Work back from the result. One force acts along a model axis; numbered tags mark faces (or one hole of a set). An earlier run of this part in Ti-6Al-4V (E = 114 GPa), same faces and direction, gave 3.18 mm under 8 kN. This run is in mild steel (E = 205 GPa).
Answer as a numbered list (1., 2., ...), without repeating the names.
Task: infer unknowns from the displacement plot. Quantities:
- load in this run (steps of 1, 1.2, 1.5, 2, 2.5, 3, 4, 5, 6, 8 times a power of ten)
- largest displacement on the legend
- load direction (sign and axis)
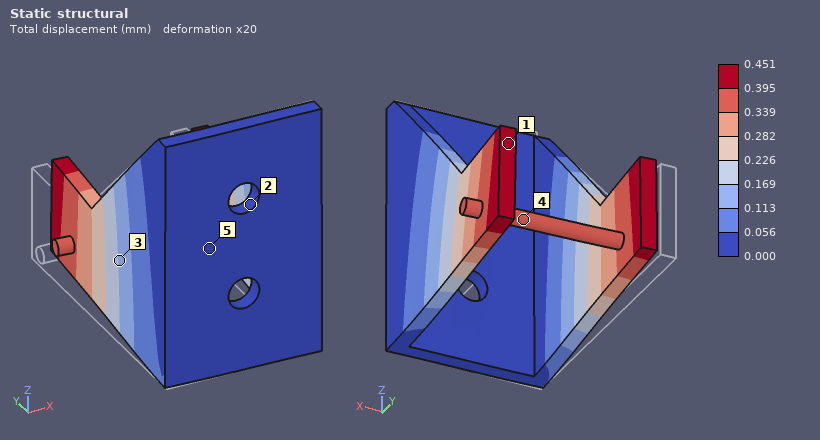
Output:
1. 2 kN
2. 0.451 mm
3. +X
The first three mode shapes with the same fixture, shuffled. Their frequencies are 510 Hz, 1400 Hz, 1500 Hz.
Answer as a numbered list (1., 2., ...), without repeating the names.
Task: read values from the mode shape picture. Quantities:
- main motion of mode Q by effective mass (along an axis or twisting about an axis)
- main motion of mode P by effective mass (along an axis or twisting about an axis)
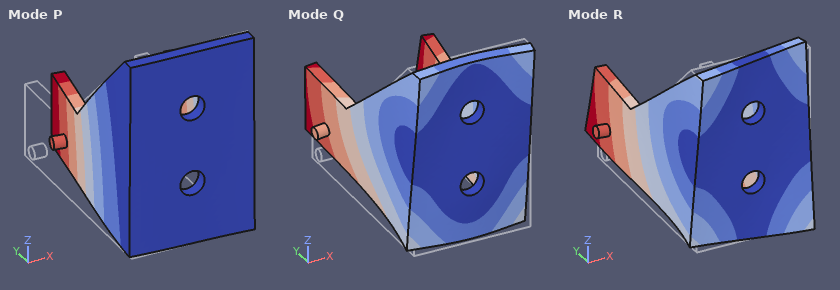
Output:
1. along Z
2. along X
